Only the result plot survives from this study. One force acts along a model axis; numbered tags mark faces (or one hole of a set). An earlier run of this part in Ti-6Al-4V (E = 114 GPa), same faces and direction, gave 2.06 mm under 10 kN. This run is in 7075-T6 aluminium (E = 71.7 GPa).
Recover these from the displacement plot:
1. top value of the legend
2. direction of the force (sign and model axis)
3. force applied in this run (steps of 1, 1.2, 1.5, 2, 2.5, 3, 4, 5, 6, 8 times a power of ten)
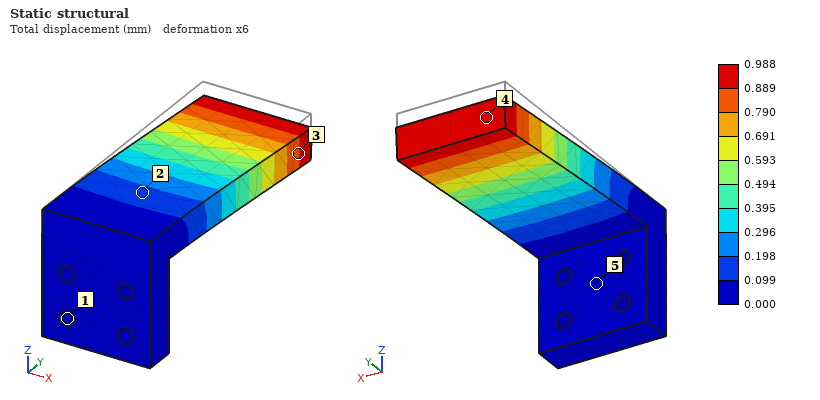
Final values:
0.988 mm
-Z
3 kN
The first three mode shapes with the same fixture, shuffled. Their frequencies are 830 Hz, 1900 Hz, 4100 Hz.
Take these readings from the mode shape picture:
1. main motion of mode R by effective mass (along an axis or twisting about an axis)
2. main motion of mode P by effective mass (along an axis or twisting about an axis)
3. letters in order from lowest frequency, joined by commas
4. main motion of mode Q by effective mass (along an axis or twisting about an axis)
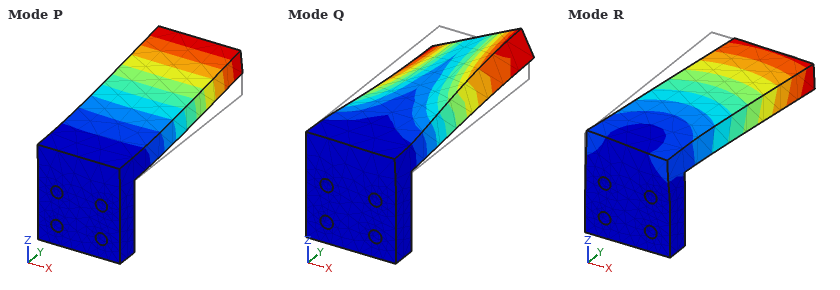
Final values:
along X
along Z
P, R, Q
twisting about Y
